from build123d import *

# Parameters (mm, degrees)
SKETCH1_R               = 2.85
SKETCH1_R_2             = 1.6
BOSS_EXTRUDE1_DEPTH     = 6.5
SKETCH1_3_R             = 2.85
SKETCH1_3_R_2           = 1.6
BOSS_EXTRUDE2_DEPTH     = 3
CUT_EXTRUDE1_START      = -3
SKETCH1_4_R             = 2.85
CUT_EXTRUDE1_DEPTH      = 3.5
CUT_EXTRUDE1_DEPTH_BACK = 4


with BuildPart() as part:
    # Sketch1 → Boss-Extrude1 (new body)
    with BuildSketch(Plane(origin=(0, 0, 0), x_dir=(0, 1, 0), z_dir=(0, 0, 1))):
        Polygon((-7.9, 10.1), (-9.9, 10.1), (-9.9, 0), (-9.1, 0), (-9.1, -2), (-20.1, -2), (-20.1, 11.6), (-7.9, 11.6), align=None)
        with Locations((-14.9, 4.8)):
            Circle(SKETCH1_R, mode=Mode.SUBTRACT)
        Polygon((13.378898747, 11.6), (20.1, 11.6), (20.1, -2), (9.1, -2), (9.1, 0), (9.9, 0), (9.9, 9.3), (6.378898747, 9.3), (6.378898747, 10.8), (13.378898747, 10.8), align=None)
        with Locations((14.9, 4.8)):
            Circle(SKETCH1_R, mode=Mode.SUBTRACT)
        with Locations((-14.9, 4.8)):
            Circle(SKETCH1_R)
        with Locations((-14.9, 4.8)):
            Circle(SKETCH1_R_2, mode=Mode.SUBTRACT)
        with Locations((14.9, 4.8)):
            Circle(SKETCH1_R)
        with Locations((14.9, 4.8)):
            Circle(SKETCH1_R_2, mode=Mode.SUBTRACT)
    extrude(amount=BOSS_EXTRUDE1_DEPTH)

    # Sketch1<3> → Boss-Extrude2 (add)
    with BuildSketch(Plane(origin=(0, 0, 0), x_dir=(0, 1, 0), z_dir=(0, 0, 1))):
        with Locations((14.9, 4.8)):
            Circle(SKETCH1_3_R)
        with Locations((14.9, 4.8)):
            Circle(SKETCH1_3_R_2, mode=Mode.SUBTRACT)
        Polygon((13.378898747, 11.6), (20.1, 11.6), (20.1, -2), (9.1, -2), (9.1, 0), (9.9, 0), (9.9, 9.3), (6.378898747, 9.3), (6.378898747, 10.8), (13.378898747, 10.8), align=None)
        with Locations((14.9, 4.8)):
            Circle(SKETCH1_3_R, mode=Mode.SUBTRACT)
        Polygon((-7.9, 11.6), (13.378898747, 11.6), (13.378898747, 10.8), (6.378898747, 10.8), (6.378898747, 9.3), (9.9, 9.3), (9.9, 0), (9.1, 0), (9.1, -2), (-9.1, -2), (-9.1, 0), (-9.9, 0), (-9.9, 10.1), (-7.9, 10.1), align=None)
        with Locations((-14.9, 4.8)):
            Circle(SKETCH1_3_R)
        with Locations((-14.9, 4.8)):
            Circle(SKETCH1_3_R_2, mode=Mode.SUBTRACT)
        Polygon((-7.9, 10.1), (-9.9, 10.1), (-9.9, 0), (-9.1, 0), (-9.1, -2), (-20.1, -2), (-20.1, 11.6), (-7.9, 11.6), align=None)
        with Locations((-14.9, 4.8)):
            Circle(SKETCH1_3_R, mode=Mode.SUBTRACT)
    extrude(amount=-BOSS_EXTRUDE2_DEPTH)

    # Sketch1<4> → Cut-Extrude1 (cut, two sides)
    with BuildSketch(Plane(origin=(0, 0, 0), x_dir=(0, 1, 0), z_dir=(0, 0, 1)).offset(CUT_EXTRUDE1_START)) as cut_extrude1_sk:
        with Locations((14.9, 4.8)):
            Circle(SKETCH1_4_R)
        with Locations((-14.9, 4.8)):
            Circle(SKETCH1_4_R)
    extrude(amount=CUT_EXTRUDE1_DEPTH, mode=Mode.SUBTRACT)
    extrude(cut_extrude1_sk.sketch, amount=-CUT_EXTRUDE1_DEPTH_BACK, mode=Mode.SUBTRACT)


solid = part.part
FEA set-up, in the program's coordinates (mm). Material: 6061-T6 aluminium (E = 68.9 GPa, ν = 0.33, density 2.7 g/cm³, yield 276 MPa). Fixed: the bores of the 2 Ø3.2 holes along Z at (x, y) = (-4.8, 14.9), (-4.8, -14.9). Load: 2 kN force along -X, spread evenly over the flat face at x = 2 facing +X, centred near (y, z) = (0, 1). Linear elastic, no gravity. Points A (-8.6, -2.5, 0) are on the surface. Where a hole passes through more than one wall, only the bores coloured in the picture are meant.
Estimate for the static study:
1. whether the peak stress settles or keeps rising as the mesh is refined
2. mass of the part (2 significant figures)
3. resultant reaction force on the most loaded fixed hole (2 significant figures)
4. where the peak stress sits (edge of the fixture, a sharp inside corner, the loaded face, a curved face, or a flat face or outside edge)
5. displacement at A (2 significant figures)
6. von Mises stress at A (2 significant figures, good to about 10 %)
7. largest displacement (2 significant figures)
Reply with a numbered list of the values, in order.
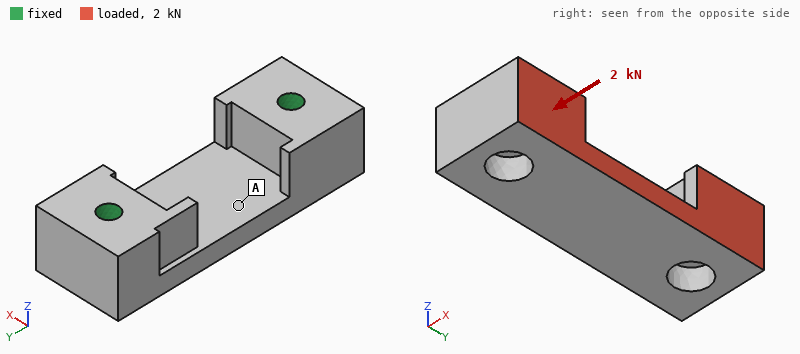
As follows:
1. keeps rising
2. 8.7 g
3. 1.0 kN
4. edge of the fixture
5. 5.8 µm
6. 6.9 MPa
7. 8.4 µm
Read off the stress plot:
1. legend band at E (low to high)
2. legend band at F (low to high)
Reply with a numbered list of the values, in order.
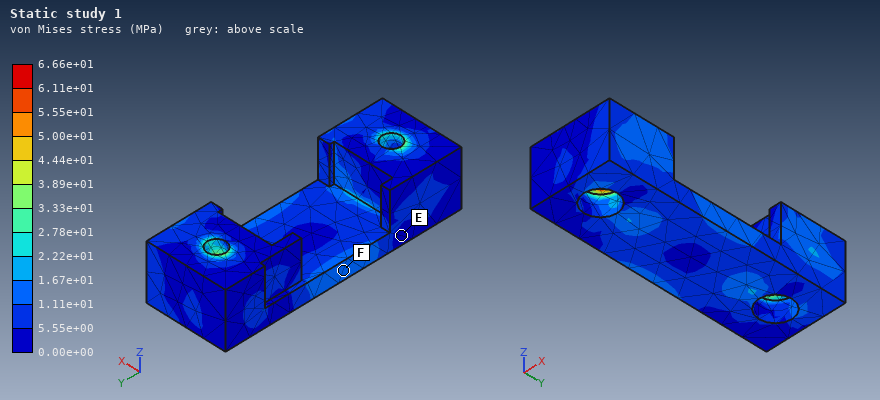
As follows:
1. 0.00e+00 to 5.55e+00 MPa
2. 1.11e+01 to 1.67e+01 MPa
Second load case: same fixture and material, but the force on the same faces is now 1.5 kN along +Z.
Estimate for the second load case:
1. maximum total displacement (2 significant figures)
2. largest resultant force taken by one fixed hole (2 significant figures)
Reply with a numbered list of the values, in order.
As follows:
1. 27 µm
2. 760 N
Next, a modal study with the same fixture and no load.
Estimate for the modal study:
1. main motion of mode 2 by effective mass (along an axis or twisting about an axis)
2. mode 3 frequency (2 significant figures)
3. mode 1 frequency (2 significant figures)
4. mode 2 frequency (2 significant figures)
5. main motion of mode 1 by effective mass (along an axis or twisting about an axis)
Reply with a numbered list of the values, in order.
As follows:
1. along X
2. 38 kHz
3. 27 kHz
4. 29 kHz
5. along Z
